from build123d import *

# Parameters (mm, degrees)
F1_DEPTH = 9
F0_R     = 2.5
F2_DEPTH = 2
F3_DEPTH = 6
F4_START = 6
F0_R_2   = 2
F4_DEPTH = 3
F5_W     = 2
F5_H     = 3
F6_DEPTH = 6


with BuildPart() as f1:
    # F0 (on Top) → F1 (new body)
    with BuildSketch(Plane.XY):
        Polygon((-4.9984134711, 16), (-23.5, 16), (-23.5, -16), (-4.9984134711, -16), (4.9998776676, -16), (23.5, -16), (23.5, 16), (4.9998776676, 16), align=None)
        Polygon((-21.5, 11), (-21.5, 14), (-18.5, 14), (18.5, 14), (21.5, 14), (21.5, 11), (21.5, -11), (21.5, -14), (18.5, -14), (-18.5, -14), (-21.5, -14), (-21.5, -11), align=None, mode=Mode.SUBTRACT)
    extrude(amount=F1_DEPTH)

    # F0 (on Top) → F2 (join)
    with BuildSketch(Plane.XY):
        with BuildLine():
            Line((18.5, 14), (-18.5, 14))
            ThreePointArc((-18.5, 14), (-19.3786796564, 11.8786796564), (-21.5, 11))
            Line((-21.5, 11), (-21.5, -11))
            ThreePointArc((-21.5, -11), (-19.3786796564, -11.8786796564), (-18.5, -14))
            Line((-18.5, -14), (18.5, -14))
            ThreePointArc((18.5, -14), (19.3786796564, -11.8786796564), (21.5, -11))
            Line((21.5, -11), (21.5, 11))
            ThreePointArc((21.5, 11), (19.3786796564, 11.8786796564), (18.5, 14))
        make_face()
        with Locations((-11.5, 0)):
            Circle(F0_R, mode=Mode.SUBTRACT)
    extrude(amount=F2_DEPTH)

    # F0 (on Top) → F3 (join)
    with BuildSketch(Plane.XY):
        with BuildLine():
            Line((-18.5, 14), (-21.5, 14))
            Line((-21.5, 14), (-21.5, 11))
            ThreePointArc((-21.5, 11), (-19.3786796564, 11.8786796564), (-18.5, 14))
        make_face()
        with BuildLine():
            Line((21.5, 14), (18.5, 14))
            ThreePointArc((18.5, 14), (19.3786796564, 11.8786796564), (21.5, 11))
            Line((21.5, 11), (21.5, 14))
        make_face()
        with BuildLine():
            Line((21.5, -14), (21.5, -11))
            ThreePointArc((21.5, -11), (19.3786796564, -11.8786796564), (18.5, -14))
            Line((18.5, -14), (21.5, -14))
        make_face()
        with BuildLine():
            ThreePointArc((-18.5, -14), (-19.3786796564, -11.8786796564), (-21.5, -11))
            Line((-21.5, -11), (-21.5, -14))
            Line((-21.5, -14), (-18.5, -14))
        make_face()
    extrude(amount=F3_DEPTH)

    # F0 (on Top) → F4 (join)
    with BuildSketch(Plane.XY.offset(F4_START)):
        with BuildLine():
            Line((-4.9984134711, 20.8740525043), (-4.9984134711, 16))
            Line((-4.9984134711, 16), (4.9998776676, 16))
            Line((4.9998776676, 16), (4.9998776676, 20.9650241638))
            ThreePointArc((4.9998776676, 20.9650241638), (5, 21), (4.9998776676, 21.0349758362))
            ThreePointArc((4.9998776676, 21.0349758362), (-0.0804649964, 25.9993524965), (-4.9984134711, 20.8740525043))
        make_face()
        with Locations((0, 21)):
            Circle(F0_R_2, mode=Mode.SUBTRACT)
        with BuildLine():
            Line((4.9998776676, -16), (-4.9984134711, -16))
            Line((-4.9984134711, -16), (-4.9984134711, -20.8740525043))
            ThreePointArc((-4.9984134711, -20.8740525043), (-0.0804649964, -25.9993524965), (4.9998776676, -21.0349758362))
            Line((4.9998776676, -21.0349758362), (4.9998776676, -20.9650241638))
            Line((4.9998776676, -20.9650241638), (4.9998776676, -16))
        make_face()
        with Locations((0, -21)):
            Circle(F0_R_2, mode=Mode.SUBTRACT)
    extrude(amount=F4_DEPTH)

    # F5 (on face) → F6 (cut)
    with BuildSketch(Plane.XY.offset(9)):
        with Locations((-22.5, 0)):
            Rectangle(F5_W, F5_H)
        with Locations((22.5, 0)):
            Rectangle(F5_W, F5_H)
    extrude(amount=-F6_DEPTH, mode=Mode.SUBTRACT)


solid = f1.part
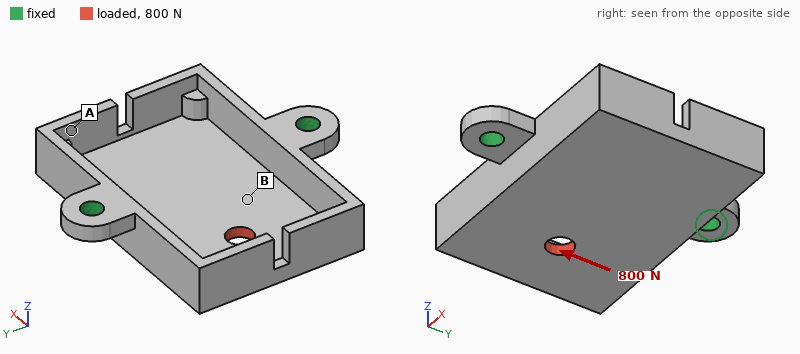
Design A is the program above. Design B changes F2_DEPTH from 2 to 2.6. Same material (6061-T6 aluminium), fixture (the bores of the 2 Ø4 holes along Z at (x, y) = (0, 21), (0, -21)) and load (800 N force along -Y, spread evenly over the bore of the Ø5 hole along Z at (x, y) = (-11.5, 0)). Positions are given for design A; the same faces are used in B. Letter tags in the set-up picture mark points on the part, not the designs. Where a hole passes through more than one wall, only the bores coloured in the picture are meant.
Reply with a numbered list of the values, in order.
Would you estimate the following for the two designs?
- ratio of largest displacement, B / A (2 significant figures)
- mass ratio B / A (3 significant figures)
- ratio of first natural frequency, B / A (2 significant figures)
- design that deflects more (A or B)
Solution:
1. 0.77
2. 1.12
3. 0.97
4. A
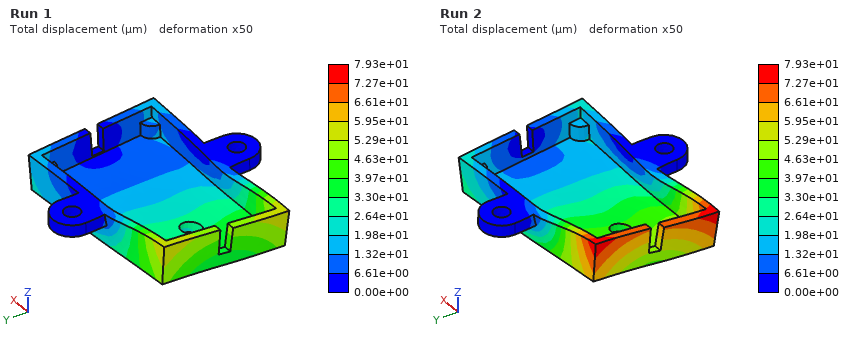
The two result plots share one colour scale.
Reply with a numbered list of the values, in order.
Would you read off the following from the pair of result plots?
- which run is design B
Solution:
1. Run 1
